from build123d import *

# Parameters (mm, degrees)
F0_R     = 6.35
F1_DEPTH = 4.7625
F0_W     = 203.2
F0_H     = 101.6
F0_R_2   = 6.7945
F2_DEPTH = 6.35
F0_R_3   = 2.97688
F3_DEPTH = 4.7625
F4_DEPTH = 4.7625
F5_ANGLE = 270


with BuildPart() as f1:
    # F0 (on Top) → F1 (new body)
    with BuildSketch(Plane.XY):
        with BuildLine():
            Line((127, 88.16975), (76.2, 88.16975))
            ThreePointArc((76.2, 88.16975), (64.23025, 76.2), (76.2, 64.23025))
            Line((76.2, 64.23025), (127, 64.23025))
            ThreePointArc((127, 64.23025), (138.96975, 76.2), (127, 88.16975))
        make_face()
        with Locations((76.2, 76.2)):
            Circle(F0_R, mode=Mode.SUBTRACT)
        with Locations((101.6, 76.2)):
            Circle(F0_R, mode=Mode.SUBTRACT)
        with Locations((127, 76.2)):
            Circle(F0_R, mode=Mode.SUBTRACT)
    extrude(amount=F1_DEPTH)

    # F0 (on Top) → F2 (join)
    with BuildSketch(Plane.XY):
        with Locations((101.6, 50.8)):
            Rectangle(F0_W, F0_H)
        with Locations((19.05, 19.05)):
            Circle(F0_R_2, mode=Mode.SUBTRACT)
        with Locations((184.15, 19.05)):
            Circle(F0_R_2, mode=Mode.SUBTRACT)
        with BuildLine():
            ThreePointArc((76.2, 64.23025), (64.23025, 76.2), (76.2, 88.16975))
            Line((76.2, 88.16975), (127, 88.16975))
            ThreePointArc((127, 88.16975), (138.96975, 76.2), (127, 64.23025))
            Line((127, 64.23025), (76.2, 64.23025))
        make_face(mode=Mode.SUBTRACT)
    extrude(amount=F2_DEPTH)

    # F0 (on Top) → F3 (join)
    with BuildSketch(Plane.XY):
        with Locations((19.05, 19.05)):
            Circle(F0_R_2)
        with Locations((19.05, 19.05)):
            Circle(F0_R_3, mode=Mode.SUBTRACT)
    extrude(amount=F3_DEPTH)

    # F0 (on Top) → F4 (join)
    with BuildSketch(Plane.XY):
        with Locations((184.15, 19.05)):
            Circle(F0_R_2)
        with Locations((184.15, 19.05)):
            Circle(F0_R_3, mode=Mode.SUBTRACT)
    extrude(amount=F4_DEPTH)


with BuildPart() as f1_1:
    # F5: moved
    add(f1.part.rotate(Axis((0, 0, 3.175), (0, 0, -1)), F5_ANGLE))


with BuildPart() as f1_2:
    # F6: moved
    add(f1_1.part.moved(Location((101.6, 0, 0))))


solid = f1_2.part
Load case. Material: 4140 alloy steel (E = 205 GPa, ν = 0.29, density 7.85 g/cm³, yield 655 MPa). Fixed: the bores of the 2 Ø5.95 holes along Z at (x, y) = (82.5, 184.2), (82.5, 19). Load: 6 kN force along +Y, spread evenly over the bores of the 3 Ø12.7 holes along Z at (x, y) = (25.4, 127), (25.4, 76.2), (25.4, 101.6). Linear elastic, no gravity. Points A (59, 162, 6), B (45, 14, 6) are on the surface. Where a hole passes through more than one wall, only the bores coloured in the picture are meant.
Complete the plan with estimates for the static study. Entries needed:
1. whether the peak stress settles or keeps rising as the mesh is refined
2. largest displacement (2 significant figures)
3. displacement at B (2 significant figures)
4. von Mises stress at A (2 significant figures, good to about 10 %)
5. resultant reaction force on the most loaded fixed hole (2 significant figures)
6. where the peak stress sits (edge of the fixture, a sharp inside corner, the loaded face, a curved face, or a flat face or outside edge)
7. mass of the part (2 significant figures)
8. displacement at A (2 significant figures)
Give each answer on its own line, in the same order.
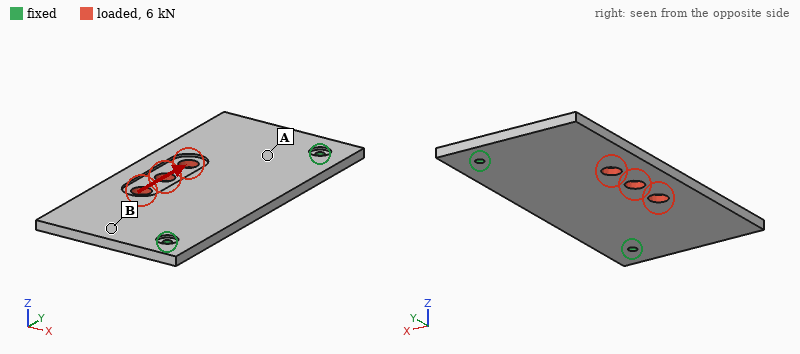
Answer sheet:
keeps rising
14 µm
7.2 µm
9.0 MPa
3.6 kN
edge of the fixture
990 g
5.3 µm
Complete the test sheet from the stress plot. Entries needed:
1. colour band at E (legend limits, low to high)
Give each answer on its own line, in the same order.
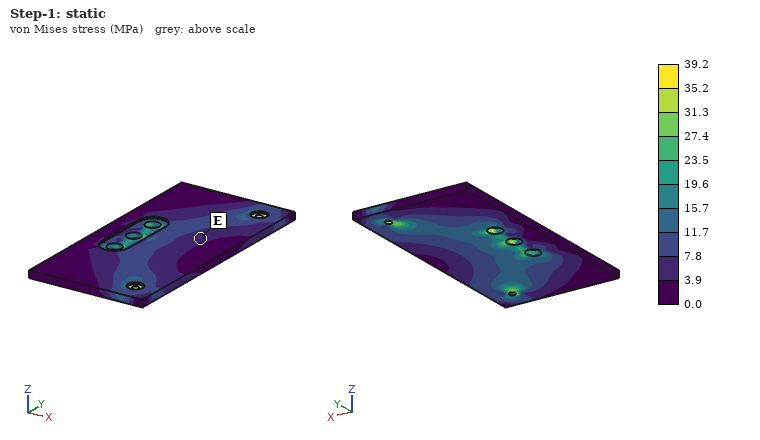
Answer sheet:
3.9 to 7.8 MPa
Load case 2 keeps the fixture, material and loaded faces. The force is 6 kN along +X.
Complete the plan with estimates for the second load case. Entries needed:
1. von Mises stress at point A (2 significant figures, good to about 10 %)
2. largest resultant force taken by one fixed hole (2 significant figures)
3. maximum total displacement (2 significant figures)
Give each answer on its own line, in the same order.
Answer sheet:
11 MPa
3.4 kN
28 µm
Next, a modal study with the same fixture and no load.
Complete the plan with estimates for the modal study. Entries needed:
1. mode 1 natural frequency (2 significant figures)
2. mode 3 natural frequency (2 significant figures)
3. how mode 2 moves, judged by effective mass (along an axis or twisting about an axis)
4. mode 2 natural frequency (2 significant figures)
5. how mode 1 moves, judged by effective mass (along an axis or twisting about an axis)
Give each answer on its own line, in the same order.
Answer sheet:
460 Hz
1000 Hz
twisting about X
890 Hz
along Z
